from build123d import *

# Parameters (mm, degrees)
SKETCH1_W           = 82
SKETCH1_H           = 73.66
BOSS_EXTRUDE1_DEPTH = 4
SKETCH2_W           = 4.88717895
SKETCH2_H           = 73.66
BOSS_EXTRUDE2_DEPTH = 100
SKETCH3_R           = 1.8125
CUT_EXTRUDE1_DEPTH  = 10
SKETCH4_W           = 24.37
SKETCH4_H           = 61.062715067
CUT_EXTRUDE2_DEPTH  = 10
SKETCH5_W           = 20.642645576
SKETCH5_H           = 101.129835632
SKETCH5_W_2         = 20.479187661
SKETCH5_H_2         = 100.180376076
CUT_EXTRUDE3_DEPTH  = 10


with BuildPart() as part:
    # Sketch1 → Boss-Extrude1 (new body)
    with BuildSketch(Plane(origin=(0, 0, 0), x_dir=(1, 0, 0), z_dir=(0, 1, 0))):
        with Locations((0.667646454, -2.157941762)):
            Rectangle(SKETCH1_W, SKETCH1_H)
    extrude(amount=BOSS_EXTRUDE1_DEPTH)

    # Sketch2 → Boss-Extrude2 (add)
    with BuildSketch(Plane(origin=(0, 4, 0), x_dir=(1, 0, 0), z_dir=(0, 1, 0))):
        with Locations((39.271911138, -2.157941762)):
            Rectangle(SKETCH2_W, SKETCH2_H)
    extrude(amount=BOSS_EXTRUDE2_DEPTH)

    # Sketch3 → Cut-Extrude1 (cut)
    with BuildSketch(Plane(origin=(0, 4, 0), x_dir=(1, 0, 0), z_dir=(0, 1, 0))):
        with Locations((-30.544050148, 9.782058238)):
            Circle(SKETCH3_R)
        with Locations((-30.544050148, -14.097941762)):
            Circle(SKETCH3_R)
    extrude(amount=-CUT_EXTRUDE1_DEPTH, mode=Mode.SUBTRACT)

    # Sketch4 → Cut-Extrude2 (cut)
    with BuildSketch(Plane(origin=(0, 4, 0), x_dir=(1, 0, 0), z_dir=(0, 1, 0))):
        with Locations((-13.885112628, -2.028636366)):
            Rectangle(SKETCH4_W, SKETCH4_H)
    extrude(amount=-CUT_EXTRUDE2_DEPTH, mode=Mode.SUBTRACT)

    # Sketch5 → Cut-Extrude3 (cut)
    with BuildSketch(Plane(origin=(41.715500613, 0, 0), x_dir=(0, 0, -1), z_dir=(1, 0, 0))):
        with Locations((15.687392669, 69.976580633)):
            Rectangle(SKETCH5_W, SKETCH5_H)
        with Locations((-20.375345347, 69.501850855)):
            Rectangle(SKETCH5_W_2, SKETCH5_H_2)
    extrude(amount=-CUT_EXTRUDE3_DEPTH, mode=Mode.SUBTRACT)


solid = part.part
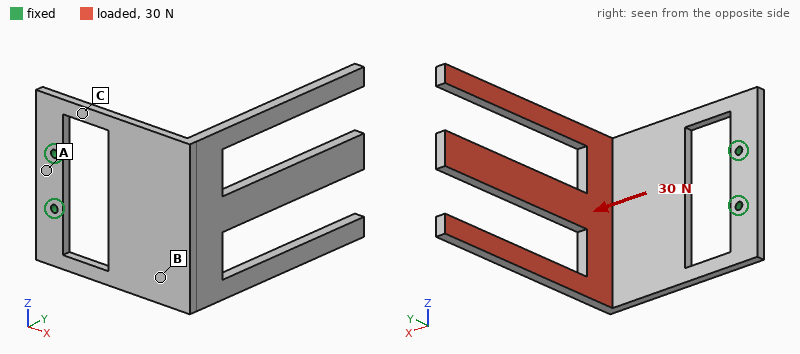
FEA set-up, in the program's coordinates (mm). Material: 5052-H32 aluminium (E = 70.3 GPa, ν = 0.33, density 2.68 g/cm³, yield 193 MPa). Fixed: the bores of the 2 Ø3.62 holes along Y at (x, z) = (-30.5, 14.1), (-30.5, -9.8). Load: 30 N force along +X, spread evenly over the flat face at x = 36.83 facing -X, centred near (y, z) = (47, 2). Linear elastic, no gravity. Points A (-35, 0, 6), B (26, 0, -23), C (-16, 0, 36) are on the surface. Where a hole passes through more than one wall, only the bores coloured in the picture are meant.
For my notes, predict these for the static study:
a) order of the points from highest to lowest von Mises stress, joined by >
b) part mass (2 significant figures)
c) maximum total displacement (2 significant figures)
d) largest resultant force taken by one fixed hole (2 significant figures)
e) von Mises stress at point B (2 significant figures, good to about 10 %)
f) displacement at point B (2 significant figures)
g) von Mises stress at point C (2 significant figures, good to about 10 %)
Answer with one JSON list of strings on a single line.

["C > B > A", "99 g", "1.6 mm", "23 N", "6.5 MPa", "0.50 mm", "40 MPa"]
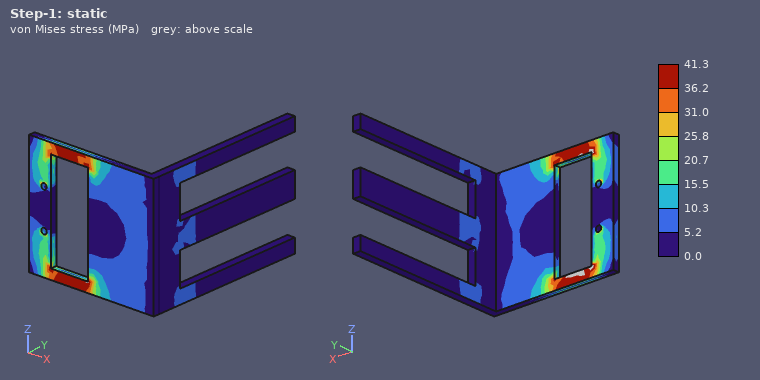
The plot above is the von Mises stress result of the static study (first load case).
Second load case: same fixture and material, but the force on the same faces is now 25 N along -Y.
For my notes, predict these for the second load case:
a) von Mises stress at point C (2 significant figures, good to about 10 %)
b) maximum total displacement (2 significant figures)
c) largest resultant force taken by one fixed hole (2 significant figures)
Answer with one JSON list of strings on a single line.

["39 MPa", "1.4 mm", "13 N"]
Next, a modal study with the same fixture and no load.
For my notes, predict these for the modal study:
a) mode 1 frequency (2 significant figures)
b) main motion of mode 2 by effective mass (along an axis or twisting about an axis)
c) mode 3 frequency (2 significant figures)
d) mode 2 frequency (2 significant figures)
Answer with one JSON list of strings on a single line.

["87 Hz", "along Z", "380 Hz", "220 Hz"]
